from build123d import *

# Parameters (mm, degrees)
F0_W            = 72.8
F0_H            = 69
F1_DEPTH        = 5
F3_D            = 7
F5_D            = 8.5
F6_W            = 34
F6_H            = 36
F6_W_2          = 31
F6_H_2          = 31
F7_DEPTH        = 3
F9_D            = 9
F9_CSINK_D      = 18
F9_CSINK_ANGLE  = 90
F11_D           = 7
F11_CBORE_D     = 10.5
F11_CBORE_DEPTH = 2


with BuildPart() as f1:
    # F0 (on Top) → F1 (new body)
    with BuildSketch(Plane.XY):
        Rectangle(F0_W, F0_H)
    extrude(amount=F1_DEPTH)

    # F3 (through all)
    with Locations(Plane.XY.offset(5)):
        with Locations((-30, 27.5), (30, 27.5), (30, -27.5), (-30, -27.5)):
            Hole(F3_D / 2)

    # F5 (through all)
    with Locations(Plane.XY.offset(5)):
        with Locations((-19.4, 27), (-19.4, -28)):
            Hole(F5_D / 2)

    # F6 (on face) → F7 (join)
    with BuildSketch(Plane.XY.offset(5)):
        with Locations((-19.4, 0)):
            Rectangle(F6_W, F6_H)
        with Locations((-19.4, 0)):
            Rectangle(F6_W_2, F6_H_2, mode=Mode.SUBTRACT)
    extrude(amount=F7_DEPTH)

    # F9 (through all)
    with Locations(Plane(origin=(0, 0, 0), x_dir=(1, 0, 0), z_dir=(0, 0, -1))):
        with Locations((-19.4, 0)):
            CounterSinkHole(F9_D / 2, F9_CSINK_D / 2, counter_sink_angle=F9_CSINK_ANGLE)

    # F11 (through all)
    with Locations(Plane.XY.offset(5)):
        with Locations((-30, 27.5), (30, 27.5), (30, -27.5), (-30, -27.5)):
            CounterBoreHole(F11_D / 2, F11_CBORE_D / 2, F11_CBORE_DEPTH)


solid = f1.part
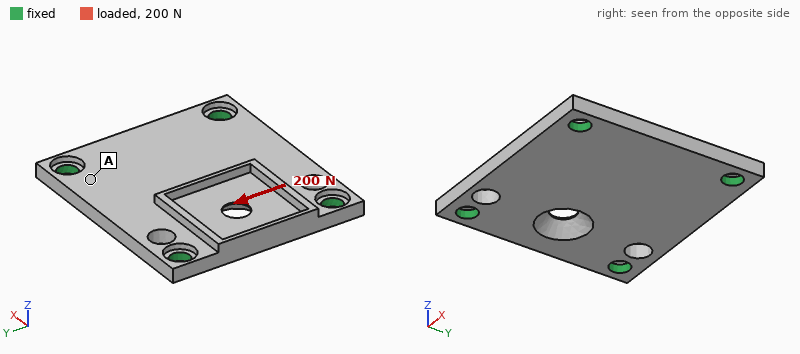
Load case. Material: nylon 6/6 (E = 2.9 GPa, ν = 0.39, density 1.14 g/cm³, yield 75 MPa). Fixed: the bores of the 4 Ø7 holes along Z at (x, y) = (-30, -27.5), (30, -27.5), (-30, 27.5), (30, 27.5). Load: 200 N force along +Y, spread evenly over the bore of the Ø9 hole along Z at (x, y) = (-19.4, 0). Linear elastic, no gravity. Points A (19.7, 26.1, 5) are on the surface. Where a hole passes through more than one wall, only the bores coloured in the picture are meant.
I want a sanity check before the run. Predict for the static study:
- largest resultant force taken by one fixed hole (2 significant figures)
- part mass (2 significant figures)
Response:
80 N
27 g
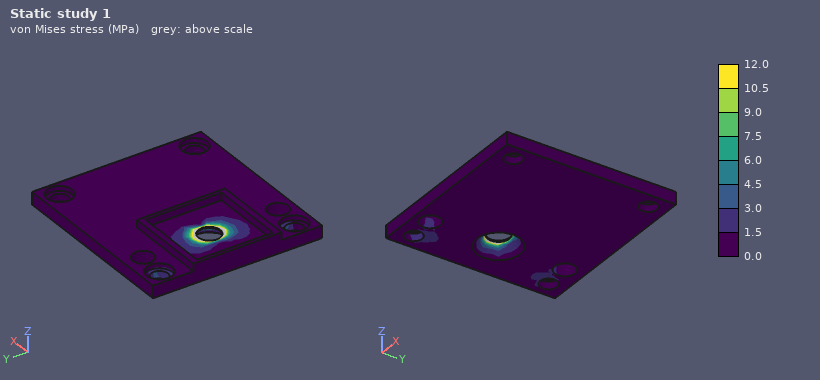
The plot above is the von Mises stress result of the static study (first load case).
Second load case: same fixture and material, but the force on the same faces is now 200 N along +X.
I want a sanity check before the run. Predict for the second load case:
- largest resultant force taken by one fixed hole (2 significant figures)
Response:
60 N
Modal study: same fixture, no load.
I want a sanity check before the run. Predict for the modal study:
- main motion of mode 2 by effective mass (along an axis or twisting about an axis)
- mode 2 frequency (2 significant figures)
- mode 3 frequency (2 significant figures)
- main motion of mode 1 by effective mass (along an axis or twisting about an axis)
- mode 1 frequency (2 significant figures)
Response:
twisting about X
2300 Hz
2700 Hz
along Z
1600 Hz
